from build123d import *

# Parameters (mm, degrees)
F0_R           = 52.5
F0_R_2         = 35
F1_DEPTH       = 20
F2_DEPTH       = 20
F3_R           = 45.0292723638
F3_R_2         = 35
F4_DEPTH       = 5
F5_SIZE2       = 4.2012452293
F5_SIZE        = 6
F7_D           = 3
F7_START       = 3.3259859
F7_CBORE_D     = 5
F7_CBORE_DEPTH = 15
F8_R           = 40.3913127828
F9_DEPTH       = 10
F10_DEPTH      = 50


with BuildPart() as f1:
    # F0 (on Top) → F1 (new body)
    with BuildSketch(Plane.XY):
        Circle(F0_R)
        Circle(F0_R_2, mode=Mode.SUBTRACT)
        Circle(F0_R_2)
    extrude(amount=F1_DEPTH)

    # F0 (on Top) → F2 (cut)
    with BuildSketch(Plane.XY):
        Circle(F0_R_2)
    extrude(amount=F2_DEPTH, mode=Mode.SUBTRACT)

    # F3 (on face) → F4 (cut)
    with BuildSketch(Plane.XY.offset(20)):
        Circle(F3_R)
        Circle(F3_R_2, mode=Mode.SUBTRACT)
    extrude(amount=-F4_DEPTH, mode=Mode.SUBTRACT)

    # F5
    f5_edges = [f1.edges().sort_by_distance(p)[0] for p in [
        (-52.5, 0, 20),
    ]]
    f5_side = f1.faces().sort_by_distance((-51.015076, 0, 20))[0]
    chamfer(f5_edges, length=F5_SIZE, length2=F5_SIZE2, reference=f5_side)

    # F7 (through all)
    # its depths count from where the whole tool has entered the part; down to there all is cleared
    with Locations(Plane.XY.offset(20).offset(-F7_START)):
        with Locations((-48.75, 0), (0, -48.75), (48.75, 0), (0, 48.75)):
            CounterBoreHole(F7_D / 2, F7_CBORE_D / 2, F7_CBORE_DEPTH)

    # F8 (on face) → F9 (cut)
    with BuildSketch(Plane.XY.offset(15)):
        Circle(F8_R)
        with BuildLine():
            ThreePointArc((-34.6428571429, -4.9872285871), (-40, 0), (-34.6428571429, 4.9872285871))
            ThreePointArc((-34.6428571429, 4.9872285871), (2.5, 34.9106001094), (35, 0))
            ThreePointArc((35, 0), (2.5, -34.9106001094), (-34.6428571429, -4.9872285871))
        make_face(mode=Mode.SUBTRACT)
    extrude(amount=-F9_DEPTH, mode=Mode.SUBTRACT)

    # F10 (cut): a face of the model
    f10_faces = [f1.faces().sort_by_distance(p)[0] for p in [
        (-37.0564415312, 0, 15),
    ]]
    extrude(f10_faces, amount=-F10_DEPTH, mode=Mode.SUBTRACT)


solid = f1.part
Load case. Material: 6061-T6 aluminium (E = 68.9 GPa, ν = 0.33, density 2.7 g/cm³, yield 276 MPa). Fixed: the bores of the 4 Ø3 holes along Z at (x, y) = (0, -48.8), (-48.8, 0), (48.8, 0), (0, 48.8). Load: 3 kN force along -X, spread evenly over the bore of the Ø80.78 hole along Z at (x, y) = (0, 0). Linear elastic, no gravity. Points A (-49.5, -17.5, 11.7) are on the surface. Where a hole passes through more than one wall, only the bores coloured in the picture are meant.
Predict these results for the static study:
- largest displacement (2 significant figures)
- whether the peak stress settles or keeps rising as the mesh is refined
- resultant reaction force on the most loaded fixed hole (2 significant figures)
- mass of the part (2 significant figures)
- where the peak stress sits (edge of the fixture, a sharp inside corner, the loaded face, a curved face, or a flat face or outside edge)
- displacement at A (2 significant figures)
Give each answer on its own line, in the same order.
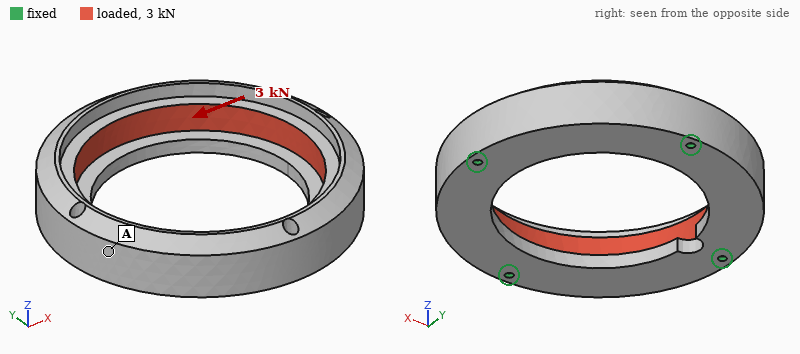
10 µm
keeps rising
1.0 kN
180 g
edge of the fixture
6.6 µm
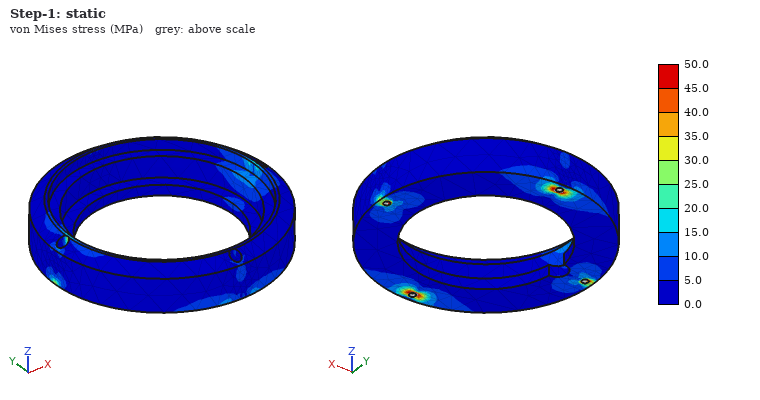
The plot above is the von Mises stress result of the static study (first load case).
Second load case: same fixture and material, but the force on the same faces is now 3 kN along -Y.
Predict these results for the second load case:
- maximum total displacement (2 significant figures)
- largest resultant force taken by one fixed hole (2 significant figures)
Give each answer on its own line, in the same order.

10 µm
1.0 kN
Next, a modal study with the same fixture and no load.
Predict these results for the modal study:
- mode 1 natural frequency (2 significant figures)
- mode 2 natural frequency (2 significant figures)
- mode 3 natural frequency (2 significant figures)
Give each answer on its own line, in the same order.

3700 Hz
6200 Hz
6200 Hz
